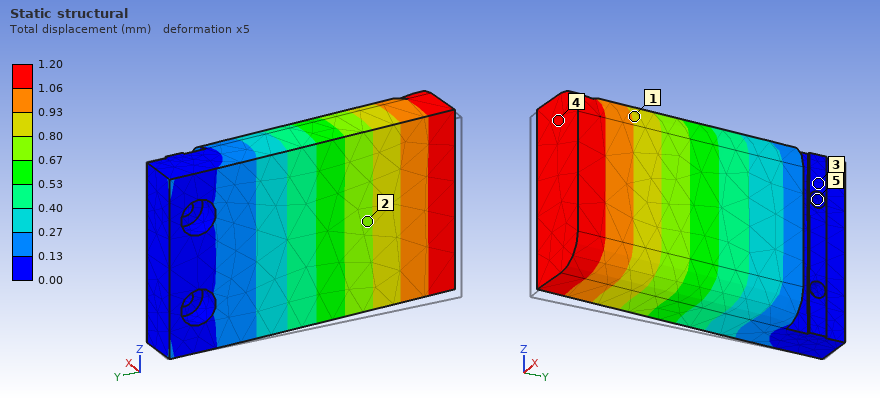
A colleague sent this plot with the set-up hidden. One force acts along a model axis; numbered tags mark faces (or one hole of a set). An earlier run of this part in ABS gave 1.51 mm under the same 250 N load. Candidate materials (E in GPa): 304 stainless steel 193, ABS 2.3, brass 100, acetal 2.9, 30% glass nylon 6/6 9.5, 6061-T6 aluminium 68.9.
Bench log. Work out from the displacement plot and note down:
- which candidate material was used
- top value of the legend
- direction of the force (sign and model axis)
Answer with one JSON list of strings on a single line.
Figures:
["acetal", "1.20 mm", "+X"]
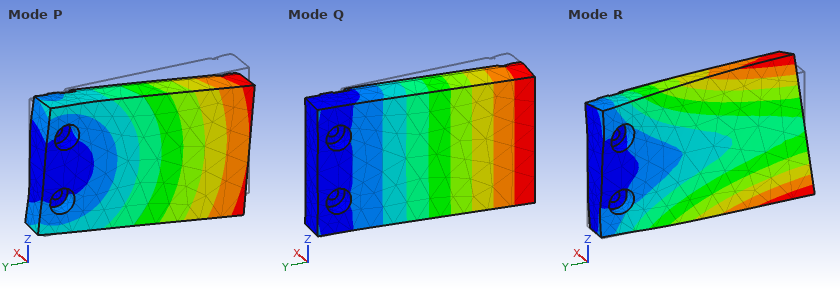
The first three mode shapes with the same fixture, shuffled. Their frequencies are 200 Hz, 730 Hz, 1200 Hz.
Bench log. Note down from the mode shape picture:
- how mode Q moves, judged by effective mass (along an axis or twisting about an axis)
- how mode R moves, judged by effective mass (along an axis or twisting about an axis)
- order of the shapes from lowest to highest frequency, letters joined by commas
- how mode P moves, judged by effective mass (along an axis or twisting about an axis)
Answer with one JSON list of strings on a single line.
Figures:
["along X", "twisting about Y", "Q, P, R", "along Z"]
